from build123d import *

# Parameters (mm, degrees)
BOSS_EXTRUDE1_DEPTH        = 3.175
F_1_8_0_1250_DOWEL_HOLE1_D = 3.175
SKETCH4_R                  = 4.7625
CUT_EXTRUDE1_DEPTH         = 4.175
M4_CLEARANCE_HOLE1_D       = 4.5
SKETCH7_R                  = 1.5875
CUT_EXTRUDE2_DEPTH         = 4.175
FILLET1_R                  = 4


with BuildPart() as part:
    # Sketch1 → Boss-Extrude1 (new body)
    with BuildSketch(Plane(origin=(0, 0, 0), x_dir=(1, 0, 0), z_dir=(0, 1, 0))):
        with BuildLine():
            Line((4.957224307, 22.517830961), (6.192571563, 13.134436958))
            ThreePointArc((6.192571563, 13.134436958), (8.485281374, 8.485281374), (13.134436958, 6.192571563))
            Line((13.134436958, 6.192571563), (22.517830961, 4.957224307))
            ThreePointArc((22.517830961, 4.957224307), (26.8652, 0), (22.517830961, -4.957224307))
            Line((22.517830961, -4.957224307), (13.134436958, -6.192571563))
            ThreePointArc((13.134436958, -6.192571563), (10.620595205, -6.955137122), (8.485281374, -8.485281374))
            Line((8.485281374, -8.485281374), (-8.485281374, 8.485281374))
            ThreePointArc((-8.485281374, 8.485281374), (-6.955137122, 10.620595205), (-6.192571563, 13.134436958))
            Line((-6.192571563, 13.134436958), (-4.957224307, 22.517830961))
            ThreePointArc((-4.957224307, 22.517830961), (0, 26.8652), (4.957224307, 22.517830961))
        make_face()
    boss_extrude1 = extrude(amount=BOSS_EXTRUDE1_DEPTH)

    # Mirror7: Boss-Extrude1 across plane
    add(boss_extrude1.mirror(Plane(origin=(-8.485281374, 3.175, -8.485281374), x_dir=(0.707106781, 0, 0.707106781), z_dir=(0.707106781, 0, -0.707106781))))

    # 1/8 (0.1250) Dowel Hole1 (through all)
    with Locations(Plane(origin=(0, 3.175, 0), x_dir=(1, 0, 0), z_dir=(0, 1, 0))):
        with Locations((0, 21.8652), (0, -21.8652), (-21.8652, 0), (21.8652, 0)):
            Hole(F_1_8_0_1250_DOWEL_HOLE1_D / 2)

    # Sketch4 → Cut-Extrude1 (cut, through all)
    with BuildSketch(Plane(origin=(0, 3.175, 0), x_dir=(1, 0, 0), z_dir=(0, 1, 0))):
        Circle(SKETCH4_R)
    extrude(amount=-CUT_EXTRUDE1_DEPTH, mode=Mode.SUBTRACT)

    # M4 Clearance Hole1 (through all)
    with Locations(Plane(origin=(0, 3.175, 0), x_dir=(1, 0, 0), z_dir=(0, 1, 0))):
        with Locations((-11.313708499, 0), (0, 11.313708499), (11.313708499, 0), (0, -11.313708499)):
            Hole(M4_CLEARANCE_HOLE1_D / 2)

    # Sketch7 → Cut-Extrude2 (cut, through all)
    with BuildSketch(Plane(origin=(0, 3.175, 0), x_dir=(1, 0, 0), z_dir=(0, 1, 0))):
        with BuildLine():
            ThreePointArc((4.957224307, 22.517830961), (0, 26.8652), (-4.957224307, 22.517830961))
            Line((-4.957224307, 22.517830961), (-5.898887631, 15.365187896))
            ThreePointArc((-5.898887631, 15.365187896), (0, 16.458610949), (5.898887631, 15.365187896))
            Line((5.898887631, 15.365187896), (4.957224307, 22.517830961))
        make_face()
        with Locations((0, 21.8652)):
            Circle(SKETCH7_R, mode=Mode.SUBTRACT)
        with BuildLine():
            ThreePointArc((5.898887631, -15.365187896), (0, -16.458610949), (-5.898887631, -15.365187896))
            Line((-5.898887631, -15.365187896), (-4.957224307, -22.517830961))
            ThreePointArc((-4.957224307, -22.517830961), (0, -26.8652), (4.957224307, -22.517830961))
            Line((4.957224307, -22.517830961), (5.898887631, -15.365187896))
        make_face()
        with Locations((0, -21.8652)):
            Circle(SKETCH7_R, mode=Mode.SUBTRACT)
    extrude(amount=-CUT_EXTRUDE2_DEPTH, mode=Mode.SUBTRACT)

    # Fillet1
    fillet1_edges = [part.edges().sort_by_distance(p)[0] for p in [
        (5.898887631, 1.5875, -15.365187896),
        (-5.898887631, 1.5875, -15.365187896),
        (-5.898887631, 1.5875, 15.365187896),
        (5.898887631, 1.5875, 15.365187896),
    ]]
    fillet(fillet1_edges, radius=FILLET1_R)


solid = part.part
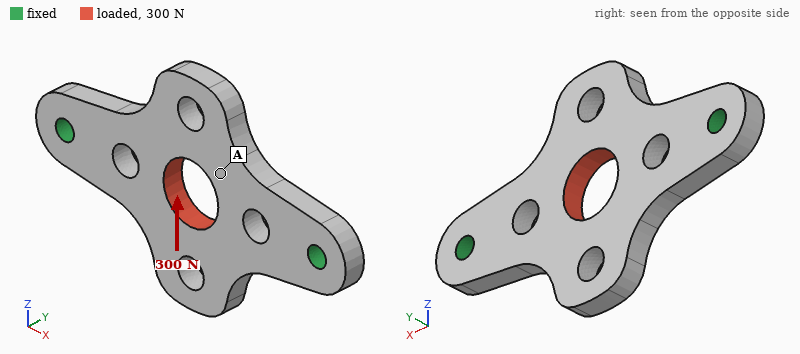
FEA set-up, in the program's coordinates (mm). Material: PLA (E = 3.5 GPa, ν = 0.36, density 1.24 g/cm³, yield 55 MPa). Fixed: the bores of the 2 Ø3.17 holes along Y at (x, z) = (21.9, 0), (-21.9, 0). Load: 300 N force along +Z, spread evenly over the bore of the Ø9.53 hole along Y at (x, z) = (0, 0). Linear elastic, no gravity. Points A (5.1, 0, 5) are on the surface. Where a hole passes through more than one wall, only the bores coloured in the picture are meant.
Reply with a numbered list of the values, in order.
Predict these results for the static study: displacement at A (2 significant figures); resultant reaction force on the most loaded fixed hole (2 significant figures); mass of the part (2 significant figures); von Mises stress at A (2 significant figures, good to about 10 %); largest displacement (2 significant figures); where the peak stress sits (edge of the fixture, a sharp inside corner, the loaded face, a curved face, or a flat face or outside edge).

1. 0.12 mm
2. 150 N
3. 2.9 g
4. 6.3 MPa
5. 0.13 mm
6. edge of the fixture
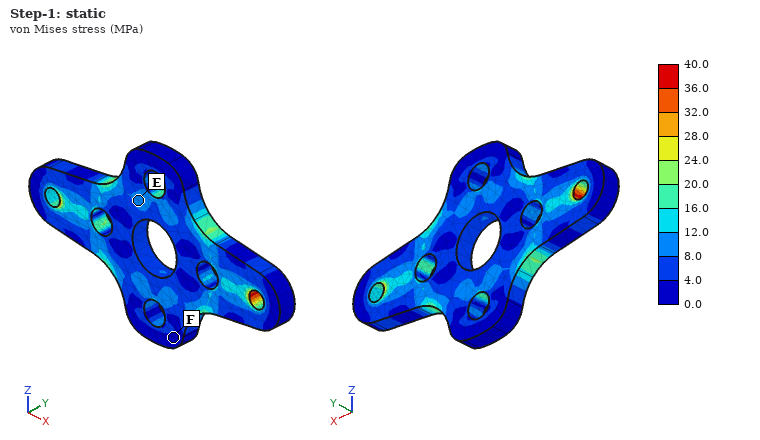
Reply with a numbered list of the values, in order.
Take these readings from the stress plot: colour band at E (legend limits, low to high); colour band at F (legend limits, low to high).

1. 8.0 to 12.0 MPa
2. 0.0 to 4.0 MPa
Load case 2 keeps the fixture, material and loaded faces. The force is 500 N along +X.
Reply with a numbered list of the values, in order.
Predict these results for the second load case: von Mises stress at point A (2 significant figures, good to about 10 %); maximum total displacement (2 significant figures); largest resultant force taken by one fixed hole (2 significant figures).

1. 6.3 MPa
2. 48 µm
3. 250 N
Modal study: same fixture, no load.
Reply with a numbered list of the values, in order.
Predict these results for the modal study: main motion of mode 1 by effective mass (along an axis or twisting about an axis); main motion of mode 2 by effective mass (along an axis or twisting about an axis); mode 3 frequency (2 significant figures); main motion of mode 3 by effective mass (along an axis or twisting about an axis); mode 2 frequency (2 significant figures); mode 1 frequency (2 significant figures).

1. twisting about X
2. along Y
3. 6000 Hz
4. along Z
5. 2000 Hz
6. 1800 Hz
